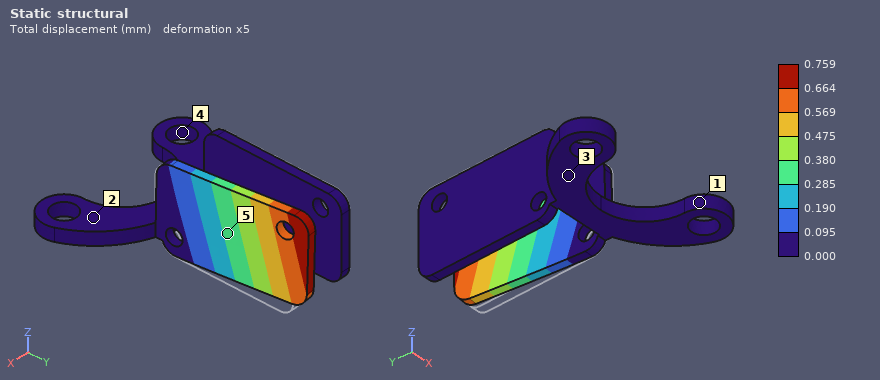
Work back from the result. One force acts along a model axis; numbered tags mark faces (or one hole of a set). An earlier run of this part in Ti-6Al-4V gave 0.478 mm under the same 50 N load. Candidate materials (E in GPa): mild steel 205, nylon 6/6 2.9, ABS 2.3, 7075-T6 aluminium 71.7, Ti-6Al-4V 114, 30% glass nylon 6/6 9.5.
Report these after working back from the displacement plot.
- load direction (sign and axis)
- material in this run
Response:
-X
7075-T6 aluminium
